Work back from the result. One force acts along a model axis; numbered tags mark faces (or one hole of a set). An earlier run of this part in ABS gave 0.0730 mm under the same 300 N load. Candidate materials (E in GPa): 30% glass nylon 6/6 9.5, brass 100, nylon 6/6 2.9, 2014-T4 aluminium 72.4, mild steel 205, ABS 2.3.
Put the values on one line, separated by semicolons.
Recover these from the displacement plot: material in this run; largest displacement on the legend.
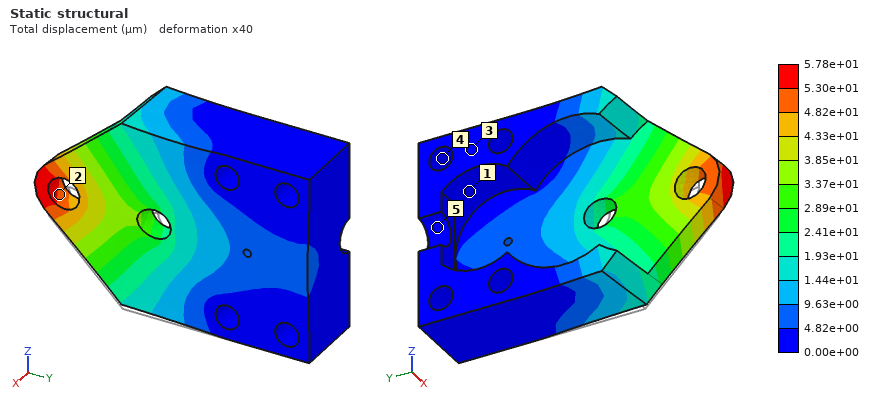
nylon 6/6; 5.78e+01 µm
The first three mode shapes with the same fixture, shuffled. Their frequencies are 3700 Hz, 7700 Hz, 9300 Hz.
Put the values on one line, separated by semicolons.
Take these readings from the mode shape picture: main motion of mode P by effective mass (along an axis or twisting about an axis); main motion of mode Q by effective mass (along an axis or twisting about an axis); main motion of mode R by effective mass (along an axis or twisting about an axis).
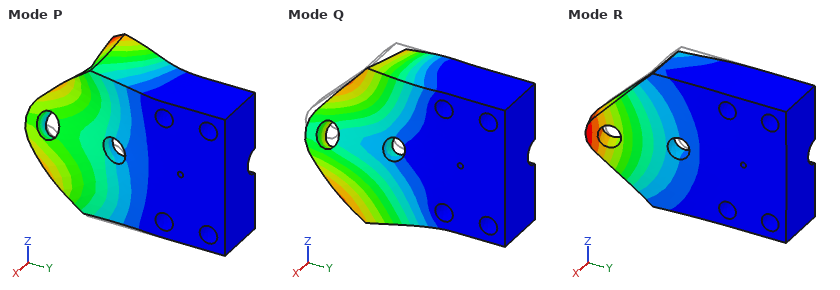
along Z; along Z; along X
